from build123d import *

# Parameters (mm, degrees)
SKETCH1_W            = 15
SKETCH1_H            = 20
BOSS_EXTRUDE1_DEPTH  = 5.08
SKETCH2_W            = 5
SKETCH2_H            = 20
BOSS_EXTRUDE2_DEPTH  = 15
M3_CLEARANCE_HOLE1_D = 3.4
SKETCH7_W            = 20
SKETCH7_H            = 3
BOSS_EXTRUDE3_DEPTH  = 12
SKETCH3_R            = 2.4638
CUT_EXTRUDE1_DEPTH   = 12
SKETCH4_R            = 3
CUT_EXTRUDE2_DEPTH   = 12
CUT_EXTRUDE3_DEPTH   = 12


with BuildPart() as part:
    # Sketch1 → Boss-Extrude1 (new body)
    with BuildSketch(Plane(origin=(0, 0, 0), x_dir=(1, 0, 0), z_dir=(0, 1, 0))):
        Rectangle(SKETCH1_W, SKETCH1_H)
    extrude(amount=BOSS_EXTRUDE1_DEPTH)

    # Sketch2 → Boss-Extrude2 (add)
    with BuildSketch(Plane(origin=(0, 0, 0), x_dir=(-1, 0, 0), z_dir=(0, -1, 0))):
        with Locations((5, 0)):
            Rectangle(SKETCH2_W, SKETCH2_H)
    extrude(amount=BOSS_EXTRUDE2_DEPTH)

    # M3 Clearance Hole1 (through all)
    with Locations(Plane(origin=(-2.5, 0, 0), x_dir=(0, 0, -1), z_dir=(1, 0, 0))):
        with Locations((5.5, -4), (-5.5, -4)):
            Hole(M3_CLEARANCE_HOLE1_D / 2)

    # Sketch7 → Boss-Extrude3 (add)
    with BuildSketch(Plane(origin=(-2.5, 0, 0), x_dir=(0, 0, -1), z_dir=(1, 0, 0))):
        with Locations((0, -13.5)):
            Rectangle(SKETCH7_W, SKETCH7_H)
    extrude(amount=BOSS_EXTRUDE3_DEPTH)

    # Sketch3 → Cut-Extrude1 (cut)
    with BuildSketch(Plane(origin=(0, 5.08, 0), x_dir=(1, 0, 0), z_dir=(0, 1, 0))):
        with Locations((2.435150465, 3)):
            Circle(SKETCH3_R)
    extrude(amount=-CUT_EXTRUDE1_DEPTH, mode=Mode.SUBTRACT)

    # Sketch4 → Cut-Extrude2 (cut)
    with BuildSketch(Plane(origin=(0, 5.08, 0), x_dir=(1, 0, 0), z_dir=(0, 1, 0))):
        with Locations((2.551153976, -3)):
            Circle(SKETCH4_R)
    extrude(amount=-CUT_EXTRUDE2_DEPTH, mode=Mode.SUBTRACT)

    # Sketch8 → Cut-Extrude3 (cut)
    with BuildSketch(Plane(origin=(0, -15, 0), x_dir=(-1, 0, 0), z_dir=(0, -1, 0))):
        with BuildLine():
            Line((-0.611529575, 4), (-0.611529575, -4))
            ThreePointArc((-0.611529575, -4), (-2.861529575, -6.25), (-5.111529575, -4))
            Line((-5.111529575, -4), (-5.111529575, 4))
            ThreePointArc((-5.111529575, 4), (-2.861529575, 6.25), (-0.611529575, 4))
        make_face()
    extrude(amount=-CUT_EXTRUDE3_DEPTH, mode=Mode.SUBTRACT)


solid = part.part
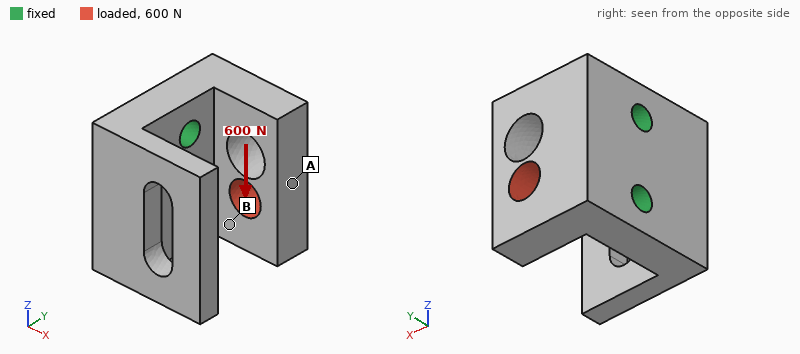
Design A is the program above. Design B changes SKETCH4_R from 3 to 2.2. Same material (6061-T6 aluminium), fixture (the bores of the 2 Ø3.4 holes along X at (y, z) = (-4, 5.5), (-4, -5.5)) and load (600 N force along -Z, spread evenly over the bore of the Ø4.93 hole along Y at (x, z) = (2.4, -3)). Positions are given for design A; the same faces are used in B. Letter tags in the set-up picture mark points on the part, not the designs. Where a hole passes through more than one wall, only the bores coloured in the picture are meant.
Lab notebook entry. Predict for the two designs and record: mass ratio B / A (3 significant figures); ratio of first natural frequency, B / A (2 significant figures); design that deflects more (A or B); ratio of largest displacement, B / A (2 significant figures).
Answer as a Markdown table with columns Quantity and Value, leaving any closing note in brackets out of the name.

| Quantity | Value |
|---|---|
| mass ratio B / A | 1.02 |
| ratio of first natural frequency, B / A | 1.0 |
| design that deflects more | A |
| ratio of largest displacement, B / A | 0.80 |
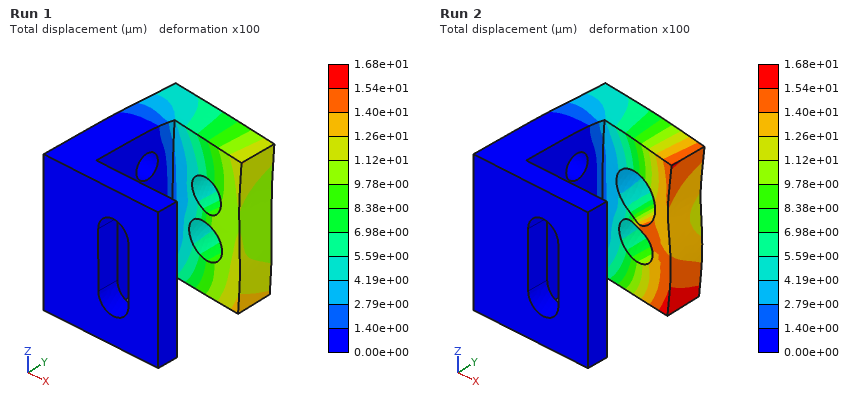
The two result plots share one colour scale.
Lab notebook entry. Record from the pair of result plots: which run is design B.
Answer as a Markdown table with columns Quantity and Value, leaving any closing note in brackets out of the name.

| Quantity | Value |
|---|---|
| which run is design B | Run 1 |
